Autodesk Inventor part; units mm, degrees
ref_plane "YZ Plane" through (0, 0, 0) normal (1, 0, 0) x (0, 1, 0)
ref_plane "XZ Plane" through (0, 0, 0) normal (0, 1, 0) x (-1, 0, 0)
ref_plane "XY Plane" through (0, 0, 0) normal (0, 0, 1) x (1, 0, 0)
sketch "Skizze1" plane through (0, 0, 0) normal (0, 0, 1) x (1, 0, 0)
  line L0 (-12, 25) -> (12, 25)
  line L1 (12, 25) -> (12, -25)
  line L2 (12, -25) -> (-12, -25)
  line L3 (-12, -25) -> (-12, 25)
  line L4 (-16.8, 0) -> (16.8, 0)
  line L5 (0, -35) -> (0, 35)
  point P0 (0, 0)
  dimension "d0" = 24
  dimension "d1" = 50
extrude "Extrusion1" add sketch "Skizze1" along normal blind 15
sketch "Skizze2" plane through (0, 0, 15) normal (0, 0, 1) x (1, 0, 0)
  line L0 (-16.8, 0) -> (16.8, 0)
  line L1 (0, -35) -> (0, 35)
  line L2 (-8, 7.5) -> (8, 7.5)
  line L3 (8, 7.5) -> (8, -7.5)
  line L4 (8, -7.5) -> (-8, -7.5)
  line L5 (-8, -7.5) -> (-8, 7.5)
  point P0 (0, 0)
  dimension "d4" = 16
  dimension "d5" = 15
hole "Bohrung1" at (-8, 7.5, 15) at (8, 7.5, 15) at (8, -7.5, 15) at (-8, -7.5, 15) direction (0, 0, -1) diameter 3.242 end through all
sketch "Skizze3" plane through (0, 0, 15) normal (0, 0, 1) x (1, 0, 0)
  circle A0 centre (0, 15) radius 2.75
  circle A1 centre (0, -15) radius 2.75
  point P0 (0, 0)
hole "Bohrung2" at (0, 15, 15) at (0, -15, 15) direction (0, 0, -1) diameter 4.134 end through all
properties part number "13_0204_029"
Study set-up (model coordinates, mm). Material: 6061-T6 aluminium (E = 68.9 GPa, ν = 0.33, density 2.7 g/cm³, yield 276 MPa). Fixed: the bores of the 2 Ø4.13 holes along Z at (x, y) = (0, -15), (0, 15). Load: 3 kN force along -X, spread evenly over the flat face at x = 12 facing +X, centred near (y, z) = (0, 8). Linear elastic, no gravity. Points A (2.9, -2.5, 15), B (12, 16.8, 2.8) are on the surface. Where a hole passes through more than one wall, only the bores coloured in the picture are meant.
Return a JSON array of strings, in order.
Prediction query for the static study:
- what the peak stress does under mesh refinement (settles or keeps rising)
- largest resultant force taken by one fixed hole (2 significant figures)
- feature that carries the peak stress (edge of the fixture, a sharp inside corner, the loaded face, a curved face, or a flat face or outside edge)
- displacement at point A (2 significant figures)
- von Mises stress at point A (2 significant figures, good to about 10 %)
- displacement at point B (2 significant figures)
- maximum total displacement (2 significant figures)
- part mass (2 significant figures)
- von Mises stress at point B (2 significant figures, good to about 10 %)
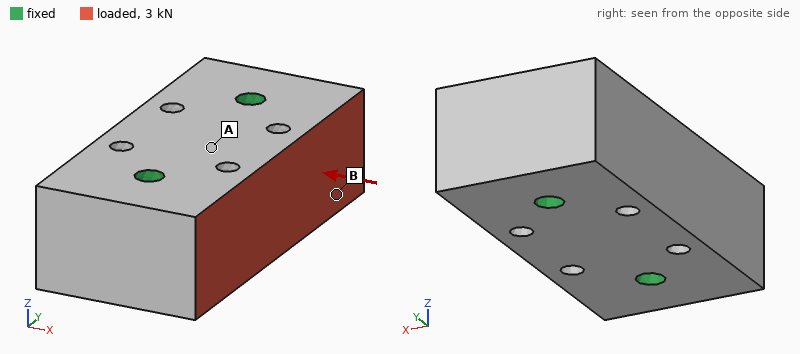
["keeps rising", "1.5 kN", "edge of the fixture", "1.2 µm", "2.5 MPa", "0.92 µm", "1.6 µm", "46 g", "5.5 MPa"]
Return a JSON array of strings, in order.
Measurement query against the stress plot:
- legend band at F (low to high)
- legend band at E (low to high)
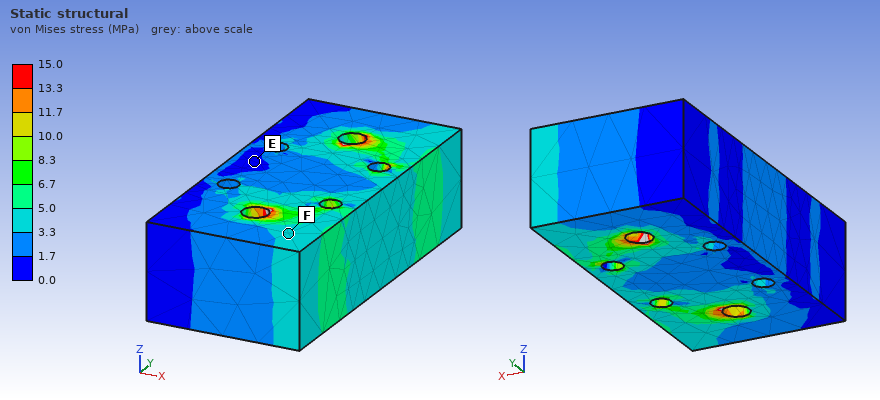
["3.3 to 5.0 MPa", "0.0 to 1.7 MPa"]
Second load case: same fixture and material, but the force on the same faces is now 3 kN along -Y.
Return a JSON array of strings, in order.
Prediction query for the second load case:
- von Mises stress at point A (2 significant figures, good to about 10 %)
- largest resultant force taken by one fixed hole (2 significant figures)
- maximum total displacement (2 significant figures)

["6.2 MPa", "1.8 kN", "5.2 µm"]
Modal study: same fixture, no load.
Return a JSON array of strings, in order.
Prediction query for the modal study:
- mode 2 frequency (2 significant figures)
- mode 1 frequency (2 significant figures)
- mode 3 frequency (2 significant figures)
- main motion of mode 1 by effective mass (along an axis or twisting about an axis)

["34 kHz", "32 kHz", "34 kHz", "twisting about Y"]
